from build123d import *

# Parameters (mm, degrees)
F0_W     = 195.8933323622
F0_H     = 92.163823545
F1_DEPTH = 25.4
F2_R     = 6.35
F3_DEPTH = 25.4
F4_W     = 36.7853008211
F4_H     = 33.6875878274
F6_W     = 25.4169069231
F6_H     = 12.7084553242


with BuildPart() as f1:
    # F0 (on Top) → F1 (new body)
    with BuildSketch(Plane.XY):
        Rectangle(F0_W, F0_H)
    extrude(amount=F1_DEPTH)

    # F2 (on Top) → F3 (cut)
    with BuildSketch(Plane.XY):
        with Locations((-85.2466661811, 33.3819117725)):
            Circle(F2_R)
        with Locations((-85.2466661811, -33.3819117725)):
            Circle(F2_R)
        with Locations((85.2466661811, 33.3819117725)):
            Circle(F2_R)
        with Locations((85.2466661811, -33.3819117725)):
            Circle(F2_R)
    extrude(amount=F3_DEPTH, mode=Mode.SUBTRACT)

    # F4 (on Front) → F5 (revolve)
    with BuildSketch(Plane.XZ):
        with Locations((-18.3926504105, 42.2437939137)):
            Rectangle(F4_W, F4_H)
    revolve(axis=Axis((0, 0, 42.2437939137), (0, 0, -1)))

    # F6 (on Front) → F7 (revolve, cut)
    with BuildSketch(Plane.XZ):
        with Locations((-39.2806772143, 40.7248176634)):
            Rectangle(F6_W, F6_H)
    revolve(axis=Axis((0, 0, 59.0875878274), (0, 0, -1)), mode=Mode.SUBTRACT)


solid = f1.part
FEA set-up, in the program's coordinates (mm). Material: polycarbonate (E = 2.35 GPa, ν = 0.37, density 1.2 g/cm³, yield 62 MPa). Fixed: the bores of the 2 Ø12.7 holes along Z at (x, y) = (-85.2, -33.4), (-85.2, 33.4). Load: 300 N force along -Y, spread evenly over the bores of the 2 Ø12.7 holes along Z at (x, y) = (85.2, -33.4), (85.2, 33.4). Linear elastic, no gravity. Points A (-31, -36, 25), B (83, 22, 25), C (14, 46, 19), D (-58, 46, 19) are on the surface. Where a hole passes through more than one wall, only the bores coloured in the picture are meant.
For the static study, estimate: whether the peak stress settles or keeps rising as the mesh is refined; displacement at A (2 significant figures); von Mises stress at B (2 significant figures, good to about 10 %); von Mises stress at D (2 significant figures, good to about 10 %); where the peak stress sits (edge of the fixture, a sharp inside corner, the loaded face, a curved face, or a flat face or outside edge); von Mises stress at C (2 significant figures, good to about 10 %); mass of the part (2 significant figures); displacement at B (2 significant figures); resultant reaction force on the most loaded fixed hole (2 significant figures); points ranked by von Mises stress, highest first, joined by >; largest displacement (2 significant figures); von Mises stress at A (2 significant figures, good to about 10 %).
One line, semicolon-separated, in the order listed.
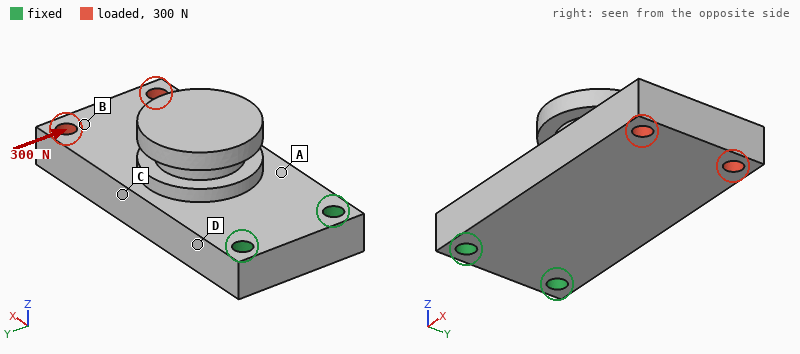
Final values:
keeps rising; 0.034 mm; 0.20 MPa; 1.2 MPa; edge of the fixture; 0.55 MPa; 680 g; 0.15 mm; 730 N; D > A > C > B; 0.17 mm; 0.82 MPa
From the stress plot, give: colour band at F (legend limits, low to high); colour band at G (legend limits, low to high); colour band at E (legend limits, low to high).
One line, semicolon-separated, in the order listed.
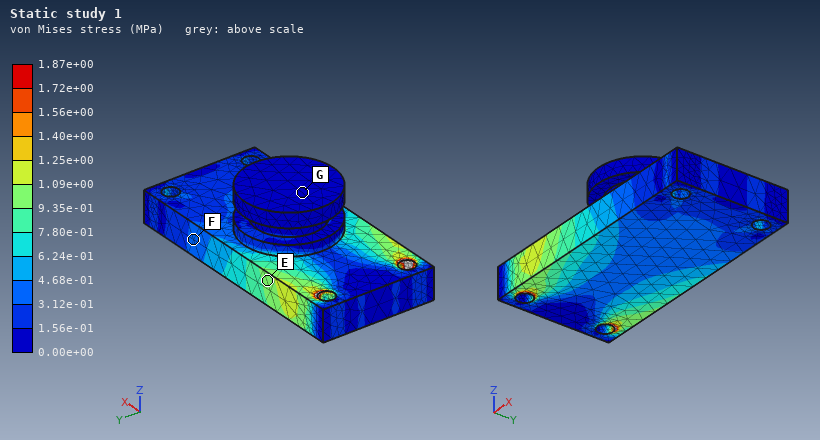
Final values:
3.12e-01 to 4.68e-01 MPa; 0.00e+00 to 1.56e-01 MPa; 9.35e-01 to 1.09e+00 MPa
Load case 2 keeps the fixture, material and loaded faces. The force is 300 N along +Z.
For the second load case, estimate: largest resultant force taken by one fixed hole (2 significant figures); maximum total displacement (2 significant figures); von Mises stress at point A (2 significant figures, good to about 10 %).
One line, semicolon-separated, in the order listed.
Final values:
150 N; 1.7 mm; 2.8 MPa
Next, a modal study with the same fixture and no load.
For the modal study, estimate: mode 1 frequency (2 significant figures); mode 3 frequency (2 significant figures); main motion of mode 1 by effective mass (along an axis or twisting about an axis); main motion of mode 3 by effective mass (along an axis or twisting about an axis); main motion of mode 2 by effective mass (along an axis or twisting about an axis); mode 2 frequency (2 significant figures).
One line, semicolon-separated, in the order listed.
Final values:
160 Hz; 650 Hz; along Z; twisting about X; along Y; 520 Hz
